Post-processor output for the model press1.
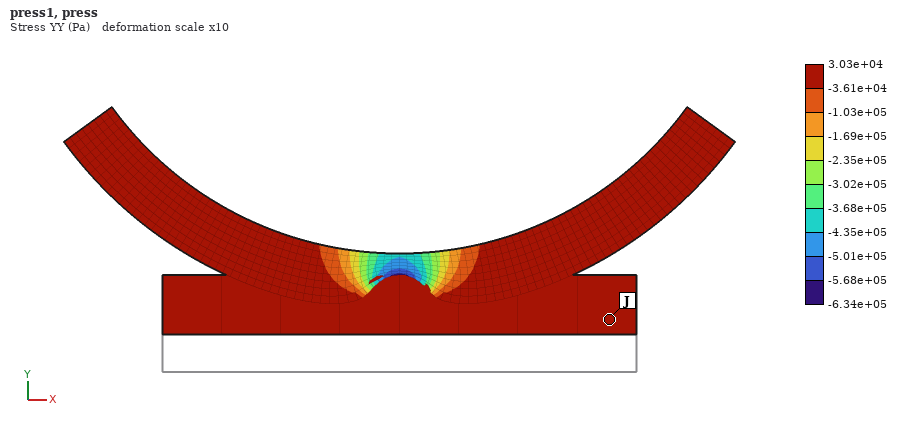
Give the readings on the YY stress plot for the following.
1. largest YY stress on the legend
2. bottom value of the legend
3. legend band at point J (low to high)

3.03e+04 Pa
-6.34e+05 Pa
-3.61e+04 to 3.03e+04 Pa
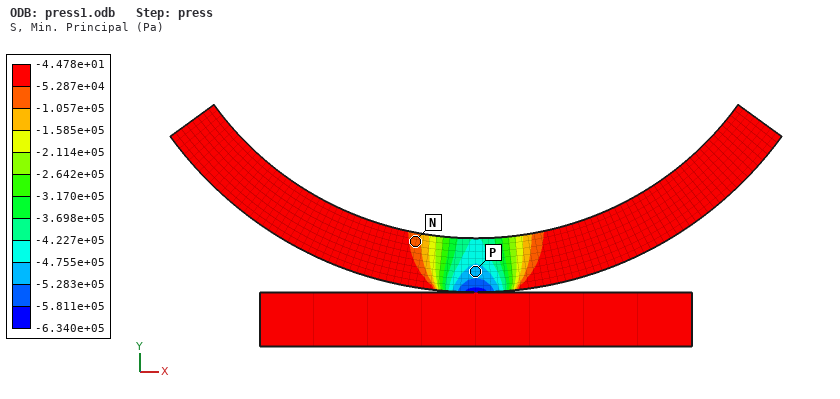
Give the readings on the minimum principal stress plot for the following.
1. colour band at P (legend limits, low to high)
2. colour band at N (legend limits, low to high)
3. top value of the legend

-5.283e+05 to -4.755e+05 Pa
-1.057e+05 to -5.287e+04 Pa
-4.478e+01 Pa
